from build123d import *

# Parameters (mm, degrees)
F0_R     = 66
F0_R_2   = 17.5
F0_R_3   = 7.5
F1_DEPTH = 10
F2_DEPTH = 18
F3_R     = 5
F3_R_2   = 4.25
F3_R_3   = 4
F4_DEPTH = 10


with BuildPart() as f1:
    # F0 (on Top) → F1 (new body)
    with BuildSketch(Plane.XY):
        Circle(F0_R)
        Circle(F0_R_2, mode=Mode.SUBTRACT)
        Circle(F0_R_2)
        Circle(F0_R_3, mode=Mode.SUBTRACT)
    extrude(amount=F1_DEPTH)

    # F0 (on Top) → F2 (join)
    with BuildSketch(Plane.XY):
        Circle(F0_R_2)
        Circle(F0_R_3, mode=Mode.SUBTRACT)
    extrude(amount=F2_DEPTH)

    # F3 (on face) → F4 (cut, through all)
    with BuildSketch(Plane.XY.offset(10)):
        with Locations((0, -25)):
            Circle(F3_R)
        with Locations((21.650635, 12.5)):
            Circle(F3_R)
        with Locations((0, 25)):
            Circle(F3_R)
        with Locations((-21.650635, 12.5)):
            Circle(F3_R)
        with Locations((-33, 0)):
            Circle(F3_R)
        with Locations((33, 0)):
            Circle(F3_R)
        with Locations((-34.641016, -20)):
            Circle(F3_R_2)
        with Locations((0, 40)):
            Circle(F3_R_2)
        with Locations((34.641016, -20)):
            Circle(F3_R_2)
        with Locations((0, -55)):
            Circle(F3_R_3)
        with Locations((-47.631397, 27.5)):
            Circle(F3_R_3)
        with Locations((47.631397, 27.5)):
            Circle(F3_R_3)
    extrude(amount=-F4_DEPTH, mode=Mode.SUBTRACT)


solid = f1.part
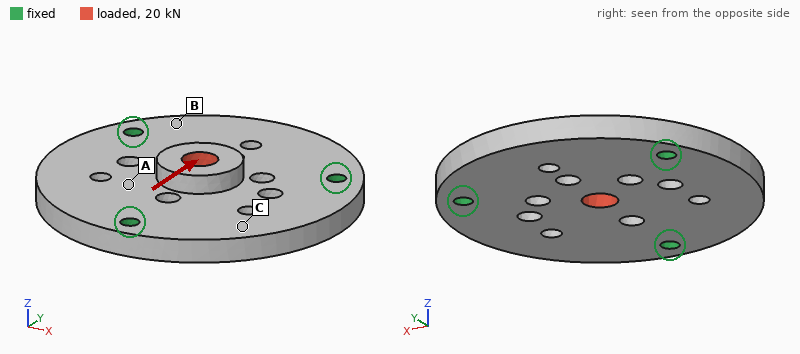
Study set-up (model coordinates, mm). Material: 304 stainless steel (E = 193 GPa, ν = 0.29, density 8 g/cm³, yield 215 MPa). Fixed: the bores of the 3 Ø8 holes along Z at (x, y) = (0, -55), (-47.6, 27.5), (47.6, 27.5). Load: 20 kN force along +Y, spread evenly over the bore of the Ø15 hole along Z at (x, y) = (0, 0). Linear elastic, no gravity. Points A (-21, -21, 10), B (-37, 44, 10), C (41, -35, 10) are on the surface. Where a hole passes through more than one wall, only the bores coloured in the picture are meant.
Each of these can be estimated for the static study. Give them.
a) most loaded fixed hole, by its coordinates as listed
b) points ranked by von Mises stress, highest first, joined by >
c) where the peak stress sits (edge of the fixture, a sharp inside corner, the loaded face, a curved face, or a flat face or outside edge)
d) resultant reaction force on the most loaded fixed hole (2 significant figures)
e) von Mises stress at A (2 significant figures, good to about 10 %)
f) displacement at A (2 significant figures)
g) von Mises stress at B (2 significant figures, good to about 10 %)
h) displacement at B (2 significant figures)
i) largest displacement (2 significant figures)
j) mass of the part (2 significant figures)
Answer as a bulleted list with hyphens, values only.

- (0, -55)
- A > B > C
- a curved face
- 7.8 kN
- 26 MPa
- 6.4 µm
- 14 MPa
- 3.3 µm
- 15 µm
- 1.1 kg
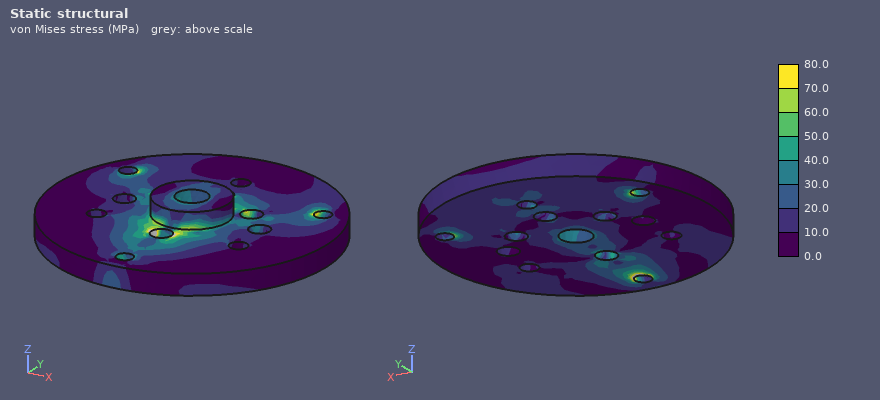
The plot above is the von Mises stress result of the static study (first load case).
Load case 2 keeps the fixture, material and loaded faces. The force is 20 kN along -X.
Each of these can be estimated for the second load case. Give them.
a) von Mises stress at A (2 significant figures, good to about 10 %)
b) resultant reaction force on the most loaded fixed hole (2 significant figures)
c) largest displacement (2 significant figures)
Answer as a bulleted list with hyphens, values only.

- 17 MPa
- 7.1 kN
- 15 µm
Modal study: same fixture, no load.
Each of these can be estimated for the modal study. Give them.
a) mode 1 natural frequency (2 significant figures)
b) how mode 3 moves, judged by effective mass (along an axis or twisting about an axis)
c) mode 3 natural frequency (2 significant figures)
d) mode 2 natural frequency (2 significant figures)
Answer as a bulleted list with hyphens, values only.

- 3600 Hz
- along Z
- 3900 Hz
- 3600 Hz
